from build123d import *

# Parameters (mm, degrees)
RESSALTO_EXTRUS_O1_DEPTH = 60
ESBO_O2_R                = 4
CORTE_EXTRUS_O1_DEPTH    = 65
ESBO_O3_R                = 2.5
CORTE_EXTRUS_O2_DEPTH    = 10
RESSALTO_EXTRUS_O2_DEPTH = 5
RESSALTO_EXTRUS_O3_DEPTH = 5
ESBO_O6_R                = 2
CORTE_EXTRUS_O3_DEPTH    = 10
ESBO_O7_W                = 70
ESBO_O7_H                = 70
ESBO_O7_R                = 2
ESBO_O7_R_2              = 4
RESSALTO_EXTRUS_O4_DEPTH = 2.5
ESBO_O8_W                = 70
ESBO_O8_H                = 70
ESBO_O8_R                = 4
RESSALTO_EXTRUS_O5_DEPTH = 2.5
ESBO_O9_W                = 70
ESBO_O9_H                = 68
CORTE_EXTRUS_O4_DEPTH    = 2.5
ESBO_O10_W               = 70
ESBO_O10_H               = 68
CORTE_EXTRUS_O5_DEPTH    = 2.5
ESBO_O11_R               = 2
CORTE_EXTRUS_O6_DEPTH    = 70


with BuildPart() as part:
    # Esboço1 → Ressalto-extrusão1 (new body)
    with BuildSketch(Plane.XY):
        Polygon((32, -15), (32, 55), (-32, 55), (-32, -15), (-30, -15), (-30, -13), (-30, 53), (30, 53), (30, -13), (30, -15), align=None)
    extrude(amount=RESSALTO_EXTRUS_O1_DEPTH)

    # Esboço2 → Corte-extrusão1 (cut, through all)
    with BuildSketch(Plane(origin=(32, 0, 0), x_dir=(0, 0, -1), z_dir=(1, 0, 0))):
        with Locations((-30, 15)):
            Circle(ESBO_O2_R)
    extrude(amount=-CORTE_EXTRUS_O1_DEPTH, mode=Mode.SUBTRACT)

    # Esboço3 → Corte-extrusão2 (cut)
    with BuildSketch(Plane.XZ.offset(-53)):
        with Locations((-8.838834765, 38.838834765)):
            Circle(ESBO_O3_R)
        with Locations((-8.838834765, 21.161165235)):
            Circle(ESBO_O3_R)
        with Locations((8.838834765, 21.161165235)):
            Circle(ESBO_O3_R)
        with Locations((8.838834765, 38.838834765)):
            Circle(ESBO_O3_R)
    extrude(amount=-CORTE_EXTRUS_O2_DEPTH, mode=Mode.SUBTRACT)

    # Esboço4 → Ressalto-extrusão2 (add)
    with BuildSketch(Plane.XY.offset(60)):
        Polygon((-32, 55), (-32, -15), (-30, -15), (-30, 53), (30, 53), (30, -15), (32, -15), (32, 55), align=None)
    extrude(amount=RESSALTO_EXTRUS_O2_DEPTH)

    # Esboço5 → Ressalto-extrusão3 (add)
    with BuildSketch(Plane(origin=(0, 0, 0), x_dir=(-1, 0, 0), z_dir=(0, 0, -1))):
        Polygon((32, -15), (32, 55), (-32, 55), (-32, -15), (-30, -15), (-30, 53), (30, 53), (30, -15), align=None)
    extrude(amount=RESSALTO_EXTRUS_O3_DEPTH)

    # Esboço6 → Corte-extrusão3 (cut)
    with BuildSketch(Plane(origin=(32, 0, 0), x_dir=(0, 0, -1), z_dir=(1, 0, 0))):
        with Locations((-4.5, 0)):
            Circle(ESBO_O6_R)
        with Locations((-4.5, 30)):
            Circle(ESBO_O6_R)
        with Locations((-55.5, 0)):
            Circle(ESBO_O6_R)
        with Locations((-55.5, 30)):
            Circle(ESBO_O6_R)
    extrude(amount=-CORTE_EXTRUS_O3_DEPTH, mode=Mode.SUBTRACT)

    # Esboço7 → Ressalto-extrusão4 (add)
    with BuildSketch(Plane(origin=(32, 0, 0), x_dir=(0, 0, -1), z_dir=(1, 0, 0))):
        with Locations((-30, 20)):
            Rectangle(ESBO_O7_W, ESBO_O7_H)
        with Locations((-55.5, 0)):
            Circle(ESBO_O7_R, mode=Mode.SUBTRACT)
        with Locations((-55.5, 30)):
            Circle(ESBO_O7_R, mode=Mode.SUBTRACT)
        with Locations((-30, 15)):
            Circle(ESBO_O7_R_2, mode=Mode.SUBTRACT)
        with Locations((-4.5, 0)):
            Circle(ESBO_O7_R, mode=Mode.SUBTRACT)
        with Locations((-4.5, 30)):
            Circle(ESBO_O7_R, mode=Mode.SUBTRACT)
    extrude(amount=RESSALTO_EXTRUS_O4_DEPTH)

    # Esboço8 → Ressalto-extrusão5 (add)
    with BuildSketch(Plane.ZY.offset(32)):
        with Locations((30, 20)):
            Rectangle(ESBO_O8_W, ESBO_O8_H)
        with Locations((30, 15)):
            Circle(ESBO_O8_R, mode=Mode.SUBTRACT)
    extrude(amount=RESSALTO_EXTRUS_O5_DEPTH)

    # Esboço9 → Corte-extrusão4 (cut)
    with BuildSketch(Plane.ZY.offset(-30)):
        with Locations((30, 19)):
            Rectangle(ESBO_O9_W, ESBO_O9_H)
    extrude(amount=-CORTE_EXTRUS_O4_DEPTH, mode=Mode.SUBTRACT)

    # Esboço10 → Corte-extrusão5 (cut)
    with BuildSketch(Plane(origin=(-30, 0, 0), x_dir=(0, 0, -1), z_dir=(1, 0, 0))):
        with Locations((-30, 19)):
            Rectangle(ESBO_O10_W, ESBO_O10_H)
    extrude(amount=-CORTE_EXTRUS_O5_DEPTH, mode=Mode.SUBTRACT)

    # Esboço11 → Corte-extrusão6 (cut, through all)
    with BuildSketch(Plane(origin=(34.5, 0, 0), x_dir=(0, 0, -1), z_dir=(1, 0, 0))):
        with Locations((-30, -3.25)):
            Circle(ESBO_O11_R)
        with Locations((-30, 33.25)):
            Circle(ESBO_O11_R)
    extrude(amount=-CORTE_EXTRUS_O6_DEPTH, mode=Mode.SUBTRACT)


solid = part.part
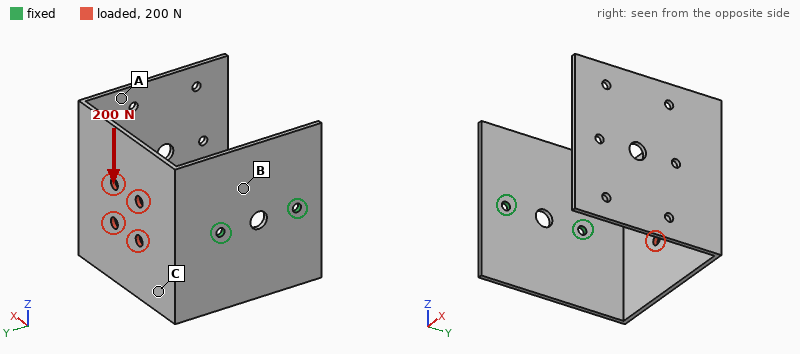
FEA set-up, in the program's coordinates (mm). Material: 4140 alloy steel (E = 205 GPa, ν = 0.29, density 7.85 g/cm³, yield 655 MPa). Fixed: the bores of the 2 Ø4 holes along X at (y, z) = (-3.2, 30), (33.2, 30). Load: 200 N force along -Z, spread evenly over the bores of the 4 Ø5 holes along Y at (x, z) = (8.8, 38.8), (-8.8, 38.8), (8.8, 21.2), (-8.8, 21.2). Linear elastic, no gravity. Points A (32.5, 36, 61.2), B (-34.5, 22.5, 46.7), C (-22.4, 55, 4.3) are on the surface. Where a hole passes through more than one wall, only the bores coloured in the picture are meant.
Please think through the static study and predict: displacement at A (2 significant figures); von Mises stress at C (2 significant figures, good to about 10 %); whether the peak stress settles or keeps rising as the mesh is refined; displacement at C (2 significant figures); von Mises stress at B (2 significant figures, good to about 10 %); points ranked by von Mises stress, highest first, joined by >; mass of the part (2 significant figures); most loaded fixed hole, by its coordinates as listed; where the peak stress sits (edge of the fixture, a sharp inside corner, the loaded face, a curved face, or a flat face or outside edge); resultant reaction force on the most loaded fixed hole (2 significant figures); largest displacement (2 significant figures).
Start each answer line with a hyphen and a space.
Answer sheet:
- 0.80 mm
- 35 MPa
- keeps rising
- 0.29 mm
- 63 MPa
- B > C > A
- 220 g
- (33.2, 30)
- edge of the fixture
- 300 N
- 0.97 mm
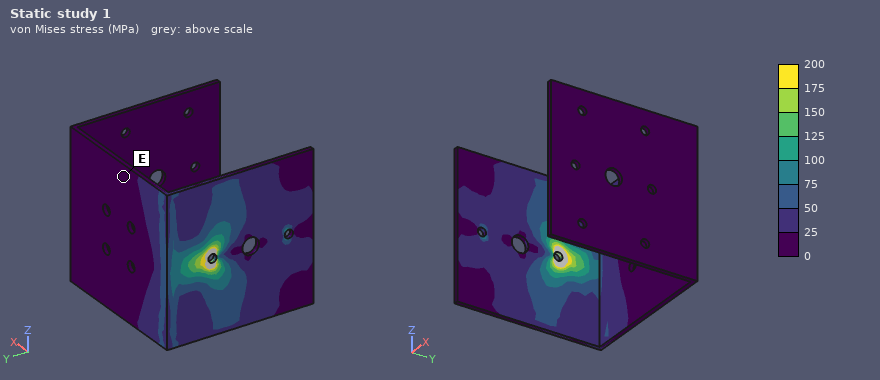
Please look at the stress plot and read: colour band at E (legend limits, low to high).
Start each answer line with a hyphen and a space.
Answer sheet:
- 0 to 25 MPa
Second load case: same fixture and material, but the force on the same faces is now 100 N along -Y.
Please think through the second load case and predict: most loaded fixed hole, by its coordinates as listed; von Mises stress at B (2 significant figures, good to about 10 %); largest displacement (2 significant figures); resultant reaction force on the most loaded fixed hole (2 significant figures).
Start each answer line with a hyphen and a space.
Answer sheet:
- (33.2, 30)
- 18 MPa
- 1.2 mm
- 87 N
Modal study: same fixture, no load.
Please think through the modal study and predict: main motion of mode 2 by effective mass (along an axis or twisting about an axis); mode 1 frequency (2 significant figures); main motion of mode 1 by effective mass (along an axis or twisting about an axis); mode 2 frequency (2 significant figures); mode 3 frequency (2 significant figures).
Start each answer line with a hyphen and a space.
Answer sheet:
- along Z
- 96 Hz
- along Y
- 140 Hz
- 260 Hz
